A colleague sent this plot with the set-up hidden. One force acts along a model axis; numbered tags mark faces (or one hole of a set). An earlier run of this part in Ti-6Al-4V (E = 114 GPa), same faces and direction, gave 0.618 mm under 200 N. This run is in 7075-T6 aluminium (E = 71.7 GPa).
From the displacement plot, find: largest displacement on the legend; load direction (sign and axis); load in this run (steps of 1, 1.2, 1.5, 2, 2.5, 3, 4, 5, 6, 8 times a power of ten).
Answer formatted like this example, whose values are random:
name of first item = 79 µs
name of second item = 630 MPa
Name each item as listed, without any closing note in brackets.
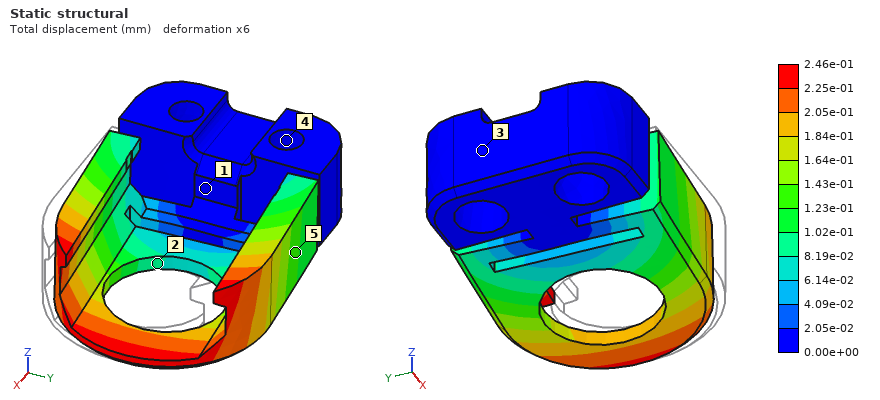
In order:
largest displacement on the legend = 2.46e-01 mm
load direction = +Y
load in this run = 50 N
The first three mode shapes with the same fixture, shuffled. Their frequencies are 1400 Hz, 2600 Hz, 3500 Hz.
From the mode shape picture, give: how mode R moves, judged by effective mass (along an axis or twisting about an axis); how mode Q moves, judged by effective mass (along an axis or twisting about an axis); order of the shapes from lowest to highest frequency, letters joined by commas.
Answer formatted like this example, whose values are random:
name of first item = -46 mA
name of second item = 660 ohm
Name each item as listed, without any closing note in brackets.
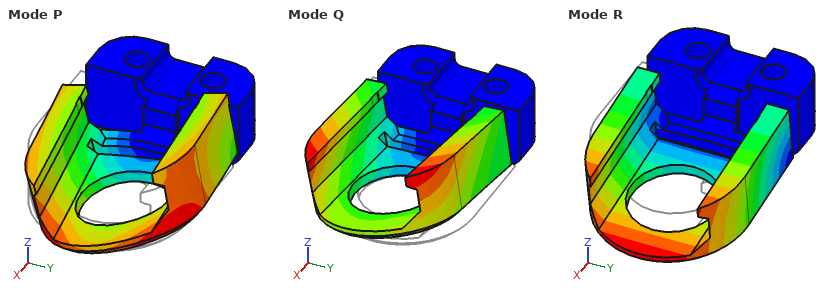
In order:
how mode R moves, judged by effective mass = along Z
how mode Q moves, judged by effective mass = along Y
order of the shapes from lowest to highest frequency, letters joined by commas = R, Q, P
